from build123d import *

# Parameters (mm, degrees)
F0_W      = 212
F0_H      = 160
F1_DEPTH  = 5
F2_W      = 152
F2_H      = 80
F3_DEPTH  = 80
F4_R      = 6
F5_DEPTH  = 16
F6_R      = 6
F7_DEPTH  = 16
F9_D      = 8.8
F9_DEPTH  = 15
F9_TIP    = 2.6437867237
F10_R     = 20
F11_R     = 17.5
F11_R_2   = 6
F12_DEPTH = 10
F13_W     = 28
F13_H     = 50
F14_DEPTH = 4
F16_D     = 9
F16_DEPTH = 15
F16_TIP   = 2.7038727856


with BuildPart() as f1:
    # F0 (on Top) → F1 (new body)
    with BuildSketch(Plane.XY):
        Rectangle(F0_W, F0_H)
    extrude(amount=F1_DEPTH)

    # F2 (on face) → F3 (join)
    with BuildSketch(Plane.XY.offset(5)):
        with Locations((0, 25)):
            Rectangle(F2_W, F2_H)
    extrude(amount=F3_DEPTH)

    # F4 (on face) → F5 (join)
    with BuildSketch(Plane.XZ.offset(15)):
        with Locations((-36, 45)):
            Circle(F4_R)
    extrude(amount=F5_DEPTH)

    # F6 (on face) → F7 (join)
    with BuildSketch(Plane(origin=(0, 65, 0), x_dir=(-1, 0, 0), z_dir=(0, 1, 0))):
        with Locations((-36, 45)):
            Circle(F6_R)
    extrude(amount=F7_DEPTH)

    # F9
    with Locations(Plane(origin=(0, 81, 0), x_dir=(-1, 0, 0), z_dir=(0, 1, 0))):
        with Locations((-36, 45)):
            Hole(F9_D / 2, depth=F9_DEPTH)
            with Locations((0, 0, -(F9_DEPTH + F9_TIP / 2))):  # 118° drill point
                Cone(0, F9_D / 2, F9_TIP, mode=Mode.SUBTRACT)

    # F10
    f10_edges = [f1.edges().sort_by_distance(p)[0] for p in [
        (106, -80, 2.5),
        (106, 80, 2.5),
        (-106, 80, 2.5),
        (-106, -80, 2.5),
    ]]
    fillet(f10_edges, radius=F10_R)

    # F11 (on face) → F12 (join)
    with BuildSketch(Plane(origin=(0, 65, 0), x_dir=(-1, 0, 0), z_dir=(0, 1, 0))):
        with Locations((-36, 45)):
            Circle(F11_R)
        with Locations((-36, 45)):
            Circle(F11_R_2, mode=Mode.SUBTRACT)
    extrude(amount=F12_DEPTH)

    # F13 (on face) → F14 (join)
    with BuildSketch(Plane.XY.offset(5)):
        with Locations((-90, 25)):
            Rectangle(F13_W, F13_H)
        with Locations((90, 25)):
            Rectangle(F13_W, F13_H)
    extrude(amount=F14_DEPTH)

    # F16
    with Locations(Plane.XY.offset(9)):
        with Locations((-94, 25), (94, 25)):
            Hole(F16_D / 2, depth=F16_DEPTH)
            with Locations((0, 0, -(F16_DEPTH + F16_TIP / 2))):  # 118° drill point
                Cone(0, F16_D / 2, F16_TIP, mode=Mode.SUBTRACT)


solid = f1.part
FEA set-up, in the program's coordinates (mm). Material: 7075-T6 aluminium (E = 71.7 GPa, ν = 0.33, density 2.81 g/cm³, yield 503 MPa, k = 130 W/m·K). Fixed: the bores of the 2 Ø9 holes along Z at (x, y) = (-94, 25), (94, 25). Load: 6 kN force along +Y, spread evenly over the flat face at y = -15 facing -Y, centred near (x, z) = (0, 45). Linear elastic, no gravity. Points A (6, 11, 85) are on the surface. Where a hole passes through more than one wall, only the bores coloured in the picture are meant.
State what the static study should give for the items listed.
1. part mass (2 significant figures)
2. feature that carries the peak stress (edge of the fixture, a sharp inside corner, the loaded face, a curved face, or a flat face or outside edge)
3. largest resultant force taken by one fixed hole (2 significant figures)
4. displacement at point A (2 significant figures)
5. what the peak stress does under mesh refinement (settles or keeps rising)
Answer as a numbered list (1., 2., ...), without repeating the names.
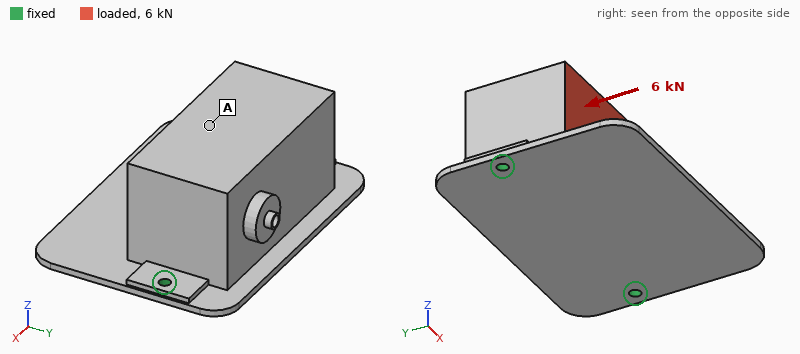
1. 3.3 kg
2. edge of the fixture
3. 3.0 kN
4. 0.50 mm
5. keeps rising
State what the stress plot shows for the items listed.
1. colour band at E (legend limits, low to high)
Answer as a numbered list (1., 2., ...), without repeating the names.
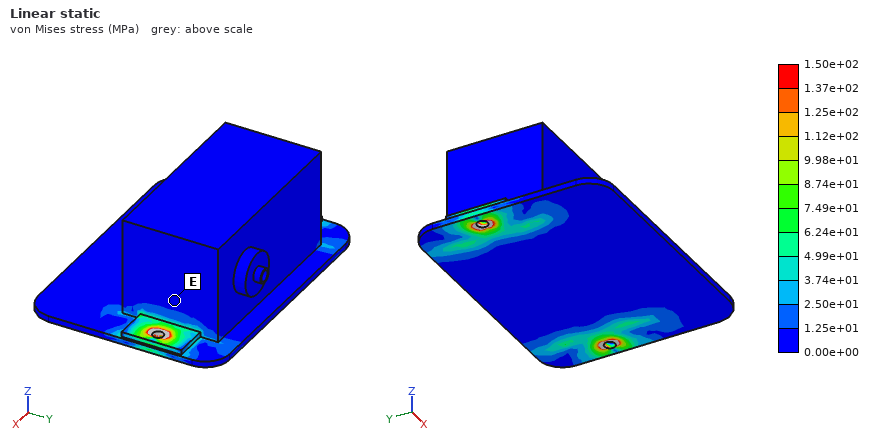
1. 0.00e+00 to 1.25e+01 MPa
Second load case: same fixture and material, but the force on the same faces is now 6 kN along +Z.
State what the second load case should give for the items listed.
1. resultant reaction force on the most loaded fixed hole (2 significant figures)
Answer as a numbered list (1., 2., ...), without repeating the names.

1. 3.3 kN
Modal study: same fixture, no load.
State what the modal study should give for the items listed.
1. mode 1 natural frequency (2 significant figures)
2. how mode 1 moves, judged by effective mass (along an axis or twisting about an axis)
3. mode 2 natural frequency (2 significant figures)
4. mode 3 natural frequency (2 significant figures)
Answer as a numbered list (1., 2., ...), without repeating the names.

1. 340 Hz
2. along Y
3. 970 Hz
4. 1100 Hz
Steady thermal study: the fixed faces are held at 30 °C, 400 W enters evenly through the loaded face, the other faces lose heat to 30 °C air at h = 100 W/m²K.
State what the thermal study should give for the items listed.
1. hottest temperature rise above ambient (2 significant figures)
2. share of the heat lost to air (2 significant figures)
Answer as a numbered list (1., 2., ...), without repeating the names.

1. 46 K
2. 68 %
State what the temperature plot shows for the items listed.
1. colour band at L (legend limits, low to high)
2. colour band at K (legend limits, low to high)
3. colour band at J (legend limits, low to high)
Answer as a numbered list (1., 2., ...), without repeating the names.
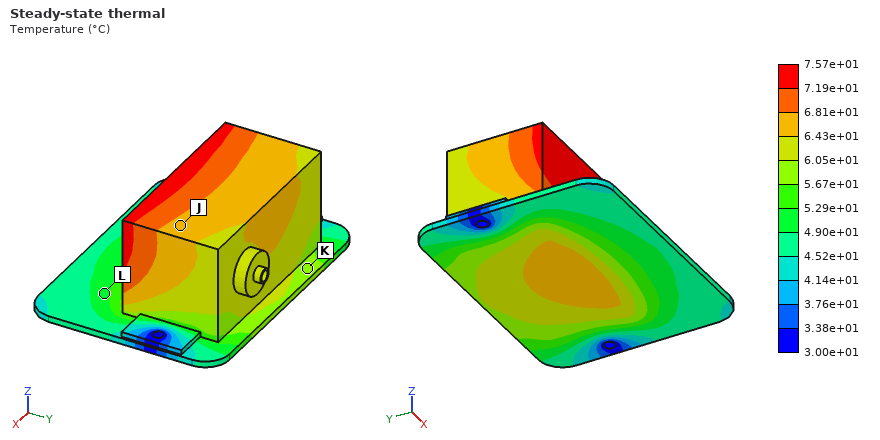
1. 4.90e+01 to 5.29e+01 °C
2. 5.67e+01 to 6.05e+01 °C
3. 6.43e+01 to 6.81e+01 °C
